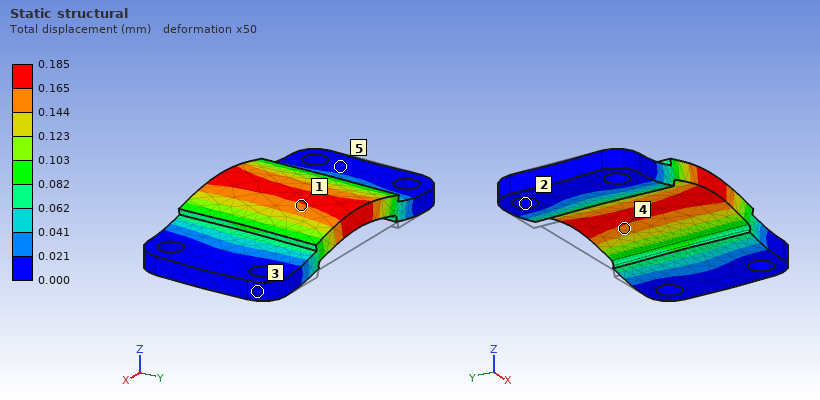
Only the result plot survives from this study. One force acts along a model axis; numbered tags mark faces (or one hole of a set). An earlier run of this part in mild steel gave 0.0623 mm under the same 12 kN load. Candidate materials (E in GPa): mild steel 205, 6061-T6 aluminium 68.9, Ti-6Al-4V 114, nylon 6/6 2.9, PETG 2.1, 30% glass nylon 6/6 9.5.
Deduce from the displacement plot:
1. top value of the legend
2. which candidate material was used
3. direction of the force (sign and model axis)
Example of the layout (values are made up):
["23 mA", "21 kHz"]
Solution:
["0.185 mm", "6061-T6 aluminium", "+Z"]
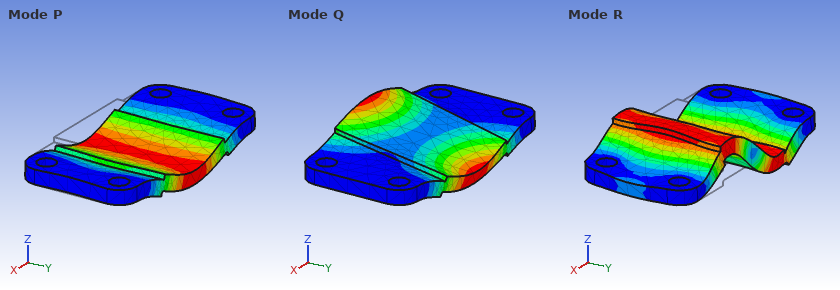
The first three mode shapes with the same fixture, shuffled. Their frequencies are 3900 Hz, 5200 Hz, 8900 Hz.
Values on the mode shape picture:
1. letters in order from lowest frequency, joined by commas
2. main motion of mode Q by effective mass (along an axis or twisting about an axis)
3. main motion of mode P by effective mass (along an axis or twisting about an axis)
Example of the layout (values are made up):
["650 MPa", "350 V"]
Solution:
["P, Q, R", "twisting about X", "along Z"]
